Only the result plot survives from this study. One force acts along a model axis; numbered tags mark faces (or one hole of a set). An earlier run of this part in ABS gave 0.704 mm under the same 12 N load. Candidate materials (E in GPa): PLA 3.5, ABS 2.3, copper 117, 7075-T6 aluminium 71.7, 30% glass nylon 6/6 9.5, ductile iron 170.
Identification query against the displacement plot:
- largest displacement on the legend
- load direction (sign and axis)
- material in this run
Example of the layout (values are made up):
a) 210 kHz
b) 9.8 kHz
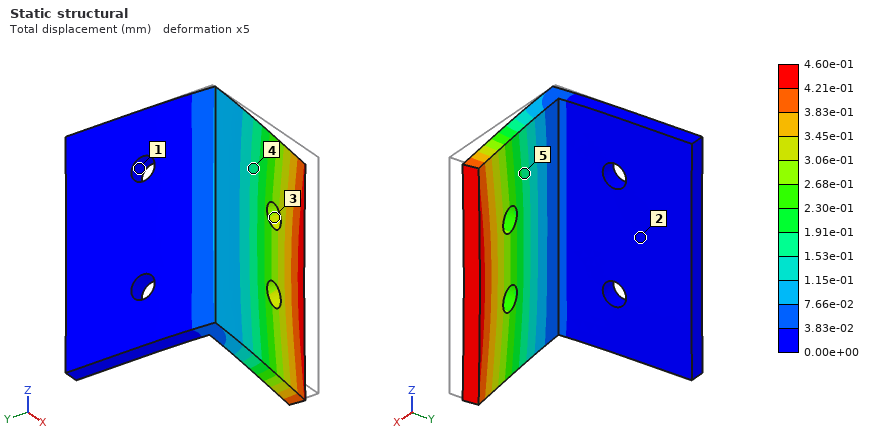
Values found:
a) 4.60e-01 mm
b) +Y
c) PLA
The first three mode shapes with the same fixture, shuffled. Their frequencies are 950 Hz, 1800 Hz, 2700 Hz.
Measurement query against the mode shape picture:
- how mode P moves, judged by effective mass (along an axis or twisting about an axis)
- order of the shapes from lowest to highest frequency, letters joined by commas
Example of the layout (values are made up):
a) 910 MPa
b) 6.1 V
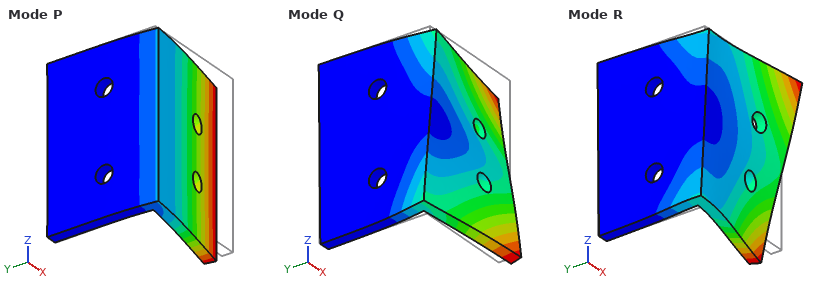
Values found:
a) along Y
b) P, Q, R
